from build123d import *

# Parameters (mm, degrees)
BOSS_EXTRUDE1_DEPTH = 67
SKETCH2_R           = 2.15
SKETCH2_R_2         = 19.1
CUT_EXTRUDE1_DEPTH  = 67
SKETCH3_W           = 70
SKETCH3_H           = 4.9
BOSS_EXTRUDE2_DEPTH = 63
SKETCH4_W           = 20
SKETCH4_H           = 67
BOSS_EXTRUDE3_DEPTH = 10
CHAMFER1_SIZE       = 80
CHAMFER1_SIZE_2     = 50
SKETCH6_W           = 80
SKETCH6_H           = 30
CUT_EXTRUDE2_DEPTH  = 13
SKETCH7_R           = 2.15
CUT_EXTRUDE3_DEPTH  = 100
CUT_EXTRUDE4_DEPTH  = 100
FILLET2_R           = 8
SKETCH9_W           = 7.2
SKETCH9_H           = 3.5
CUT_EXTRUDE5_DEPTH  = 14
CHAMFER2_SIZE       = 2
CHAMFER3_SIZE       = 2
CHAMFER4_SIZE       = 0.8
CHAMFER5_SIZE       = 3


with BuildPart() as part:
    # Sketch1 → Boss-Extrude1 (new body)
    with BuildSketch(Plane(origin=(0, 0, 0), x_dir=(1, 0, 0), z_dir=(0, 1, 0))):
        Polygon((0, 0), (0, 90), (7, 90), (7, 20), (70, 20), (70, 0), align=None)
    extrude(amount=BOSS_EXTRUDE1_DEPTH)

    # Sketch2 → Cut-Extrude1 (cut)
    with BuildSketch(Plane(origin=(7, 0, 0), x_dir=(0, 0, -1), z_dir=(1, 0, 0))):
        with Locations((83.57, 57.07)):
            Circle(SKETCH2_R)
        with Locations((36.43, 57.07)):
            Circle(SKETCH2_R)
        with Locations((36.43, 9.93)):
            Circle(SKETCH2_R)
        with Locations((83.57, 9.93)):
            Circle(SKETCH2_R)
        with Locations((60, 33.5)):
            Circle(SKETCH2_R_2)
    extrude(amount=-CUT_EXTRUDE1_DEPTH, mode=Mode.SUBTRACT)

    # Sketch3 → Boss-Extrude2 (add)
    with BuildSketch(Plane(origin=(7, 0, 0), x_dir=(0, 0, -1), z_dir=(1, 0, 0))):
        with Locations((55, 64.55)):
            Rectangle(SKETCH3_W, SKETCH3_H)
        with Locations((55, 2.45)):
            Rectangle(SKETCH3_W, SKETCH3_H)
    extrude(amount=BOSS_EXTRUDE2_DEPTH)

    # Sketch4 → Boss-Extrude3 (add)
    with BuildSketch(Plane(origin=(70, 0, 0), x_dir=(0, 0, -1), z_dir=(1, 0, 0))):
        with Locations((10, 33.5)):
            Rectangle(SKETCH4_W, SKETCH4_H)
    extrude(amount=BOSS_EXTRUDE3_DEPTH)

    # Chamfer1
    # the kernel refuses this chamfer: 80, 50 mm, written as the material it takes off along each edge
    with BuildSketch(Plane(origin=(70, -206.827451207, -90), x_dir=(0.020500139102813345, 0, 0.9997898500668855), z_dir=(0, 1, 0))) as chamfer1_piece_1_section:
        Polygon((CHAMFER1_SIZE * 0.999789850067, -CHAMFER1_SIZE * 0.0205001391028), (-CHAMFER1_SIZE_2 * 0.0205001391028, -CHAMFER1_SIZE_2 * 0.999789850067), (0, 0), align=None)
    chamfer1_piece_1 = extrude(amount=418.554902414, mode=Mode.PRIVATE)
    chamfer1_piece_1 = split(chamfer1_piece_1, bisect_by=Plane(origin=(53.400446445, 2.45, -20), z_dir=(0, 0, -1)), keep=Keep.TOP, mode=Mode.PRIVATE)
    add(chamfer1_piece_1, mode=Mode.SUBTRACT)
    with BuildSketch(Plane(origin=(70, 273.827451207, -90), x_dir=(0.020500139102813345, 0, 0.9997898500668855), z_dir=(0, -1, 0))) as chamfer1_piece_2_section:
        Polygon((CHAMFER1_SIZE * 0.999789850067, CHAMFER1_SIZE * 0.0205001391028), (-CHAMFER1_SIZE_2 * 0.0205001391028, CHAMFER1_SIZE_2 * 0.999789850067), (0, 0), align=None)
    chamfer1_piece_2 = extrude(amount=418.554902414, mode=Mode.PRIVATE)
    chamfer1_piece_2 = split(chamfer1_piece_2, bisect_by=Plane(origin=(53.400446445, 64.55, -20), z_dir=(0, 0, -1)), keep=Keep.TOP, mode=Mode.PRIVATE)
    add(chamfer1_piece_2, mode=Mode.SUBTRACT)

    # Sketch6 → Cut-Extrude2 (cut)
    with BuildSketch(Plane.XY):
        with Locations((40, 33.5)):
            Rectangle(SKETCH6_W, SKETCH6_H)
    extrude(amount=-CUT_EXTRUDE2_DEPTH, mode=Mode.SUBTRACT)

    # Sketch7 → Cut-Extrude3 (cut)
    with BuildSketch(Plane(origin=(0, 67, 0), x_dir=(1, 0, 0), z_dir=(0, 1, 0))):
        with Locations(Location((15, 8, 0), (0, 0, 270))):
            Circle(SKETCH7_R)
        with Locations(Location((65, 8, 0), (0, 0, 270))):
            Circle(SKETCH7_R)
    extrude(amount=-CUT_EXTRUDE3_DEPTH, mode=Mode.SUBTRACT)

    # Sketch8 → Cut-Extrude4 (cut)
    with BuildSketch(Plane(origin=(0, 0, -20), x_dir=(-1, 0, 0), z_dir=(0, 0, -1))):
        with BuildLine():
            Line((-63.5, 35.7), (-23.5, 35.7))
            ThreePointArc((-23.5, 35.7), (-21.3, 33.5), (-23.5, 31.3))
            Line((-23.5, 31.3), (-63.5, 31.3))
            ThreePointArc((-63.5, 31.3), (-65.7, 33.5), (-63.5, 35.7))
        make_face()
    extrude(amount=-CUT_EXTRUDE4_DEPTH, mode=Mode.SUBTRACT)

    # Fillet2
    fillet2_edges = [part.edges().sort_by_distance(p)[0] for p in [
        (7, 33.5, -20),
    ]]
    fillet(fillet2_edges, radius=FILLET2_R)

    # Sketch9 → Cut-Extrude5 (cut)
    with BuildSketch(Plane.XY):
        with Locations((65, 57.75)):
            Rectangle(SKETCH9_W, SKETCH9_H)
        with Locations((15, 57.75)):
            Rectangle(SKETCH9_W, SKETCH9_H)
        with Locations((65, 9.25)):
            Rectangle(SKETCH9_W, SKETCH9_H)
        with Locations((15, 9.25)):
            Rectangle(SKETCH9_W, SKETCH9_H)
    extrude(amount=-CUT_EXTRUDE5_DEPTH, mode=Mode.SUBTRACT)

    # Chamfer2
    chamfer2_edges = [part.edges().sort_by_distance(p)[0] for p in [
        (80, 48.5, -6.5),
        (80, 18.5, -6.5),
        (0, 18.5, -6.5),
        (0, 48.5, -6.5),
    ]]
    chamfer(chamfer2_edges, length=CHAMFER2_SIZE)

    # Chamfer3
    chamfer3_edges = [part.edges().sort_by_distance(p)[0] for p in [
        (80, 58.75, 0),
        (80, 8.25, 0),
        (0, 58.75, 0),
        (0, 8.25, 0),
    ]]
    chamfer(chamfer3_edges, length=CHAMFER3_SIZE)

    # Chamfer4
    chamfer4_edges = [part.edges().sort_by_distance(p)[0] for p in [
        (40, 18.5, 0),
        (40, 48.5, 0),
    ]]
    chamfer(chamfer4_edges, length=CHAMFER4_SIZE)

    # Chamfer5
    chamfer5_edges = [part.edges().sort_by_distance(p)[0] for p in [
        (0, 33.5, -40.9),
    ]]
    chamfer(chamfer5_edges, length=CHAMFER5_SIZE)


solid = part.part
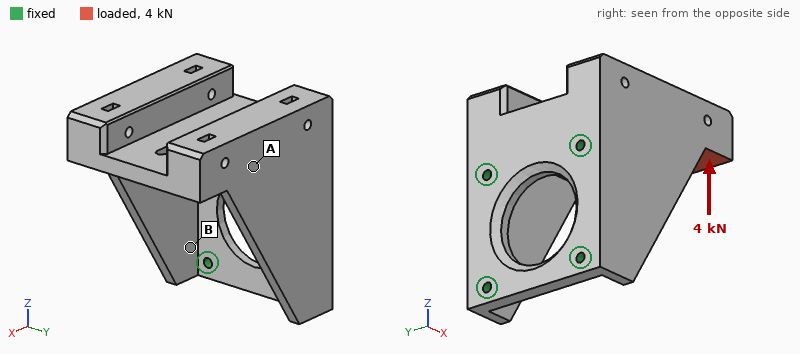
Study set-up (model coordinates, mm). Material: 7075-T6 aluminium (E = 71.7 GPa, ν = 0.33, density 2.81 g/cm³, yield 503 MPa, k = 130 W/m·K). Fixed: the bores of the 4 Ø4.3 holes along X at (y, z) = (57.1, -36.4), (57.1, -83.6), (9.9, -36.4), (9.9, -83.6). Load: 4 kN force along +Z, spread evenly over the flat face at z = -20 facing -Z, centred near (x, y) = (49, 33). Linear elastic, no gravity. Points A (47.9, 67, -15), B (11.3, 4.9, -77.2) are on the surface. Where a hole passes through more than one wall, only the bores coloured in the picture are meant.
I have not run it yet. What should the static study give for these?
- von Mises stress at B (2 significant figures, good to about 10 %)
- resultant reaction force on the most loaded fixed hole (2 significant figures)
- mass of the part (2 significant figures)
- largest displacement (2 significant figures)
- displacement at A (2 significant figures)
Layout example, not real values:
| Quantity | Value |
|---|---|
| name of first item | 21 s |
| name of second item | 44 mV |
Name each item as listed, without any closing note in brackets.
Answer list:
| Quantity | Value |
|---|---|
| von Mises stress at B | 33 MPa |
| resultant reaction force on the most loaded fixed hole | 2.2 kN |
| mass of the part | 340 g |
| largest displacement | 0.15 mm |
| displacement at A | 0.054 mm |
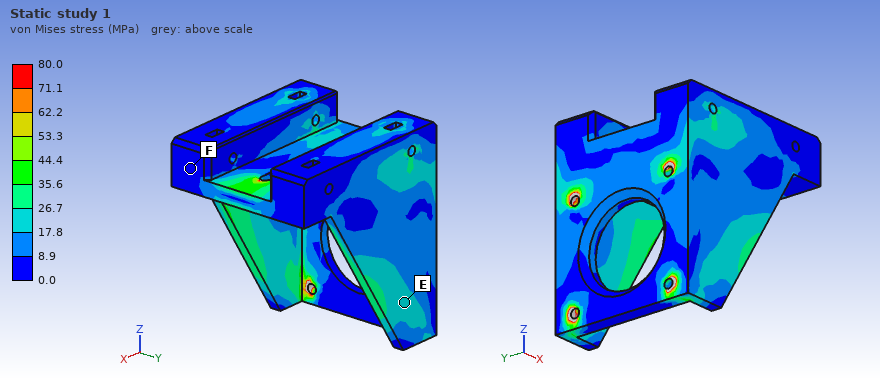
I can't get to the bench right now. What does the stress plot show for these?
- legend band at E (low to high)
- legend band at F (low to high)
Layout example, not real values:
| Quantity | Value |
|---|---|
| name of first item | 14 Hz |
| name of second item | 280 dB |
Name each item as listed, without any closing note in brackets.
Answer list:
| Quantity | Value |
|---|---|
| legend band at E | 17.8 to 26.7 MPa |
| legend band at F | 0.0 to 8.9 MPa |
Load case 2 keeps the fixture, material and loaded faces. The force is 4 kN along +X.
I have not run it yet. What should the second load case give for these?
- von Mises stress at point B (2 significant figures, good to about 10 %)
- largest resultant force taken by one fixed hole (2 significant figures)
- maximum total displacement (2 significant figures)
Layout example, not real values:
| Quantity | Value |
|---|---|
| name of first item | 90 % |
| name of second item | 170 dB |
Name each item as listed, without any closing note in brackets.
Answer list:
| Quantity | Value |
|---|---|
| von Mises stress at point B | 12 MPa |
| largest resultant force taken by one fixed hole | 2.6 kN |
| maximum total displacement | 44 µm |
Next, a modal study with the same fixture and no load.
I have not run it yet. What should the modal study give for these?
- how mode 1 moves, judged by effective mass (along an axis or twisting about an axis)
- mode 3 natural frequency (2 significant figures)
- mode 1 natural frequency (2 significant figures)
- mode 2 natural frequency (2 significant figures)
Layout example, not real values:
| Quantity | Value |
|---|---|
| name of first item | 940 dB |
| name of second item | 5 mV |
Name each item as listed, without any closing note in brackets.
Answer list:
| Quantity | Value |
|---|---|
| how mode 1 moves, judged by effective mass | along Y |
| mode 3 natural frequency | 4700 Hz |
| mode 1 natural frequency | 2200 Hz |
| mode 2 natural frequency | 2400 Hz |
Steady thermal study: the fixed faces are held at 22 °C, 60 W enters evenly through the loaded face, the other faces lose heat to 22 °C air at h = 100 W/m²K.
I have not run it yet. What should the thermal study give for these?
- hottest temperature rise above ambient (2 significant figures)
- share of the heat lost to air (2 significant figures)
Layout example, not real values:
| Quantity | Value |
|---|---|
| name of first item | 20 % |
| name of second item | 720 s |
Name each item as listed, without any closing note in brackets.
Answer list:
| Quantity | Value |
|---|---|
| hottest temperature rise above ambient | 21 K |
| share of the heat lost to air | 49 % |
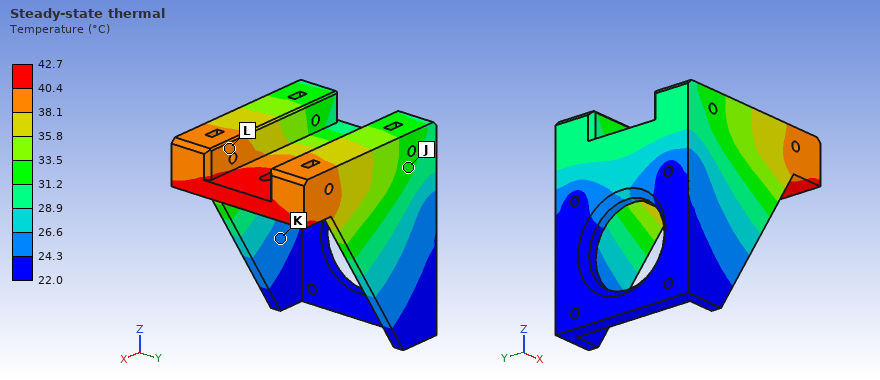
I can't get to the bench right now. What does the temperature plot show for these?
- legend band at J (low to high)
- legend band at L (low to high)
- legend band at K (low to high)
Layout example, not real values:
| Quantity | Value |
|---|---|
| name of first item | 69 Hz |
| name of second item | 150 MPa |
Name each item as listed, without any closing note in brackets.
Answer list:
| Quantity | Value |
|---|---|
| legend band at J | 31.2 to 33.5 °C |
| legend band at L | 38.1 to 40.4 °C |
| legend band at K | 24.3 to 26.6 °C |
